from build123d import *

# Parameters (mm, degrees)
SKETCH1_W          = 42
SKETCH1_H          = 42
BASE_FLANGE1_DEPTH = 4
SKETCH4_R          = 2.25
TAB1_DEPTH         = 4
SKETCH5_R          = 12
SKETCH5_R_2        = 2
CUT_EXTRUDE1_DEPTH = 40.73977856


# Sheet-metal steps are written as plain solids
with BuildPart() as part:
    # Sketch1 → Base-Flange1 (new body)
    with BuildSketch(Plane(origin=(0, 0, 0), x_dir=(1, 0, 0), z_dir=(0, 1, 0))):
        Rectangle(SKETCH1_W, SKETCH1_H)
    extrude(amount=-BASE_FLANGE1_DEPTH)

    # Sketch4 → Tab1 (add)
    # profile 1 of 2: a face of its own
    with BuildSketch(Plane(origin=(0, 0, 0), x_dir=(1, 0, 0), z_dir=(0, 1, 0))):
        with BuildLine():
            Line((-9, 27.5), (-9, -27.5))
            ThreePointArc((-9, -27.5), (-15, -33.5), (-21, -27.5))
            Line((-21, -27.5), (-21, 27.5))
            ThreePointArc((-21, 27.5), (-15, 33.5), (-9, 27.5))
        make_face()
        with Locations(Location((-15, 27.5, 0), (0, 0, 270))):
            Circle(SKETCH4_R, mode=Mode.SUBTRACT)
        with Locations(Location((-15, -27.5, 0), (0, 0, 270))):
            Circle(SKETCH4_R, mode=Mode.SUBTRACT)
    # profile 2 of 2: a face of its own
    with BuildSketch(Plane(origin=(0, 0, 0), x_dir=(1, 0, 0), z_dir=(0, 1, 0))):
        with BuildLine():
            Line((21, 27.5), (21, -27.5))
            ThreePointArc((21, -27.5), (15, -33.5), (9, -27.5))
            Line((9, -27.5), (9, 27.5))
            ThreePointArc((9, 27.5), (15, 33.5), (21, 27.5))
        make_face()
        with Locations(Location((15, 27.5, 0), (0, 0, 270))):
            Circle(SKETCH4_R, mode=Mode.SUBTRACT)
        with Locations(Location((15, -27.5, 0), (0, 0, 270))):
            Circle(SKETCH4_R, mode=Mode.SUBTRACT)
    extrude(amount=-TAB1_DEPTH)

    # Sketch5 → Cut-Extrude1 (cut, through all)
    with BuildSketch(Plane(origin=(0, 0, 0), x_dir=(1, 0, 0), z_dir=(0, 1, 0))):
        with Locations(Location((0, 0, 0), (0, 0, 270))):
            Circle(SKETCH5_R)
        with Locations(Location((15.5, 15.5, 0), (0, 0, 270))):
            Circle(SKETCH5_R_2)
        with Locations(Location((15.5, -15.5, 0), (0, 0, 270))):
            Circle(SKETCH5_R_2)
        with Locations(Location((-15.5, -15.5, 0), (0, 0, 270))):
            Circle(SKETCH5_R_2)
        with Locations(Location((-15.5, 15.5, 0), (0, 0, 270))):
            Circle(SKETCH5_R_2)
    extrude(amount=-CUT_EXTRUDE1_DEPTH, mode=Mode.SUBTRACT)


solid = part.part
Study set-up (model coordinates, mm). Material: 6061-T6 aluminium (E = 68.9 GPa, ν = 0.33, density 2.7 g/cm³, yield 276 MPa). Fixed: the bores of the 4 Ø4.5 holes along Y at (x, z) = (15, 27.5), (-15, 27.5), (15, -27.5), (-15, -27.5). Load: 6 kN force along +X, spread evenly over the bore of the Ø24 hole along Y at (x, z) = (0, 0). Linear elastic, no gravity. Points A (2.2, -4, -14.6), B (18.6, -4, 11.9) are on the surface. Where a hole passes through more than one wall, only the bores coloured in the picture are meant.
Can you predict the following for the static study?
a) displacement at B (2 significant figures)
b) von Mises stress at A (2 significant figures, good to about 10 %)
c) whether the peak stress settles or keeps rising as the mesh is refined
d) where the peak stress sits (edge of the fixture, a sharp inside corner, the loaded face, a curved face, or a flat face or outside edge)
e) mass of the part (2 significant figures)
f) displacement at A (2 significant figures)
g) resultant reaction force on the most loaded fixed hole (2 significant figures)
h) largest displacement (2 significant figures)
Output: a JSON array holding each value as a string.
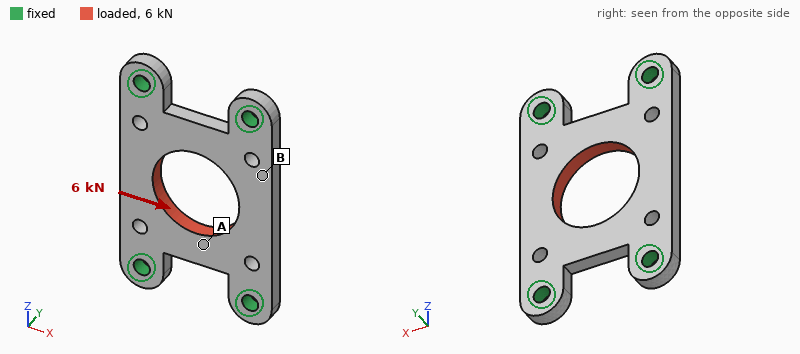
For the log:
["31 µm", "76 MPa", "keeps rising", "edge of the fixture", "19 g", "26 µm", "1.6 kN", "45 µm"]
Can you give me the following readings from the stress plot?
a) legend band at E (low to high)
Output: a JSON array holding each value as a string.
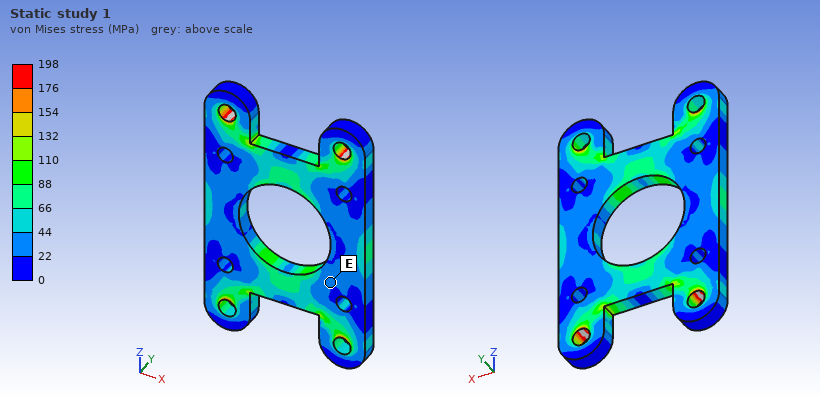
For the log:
["22 to 44 MPa"]
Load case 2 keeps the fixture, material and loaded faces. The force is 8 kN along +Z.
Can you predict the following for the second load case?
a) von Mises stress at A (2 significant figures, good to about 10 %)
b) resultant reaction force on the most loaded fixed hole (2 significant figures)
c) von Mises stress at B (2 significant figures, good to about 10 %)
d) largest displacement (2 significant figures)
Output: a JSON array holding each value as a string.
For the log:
["25 MPa", "2.1 kN", "32 MPa", "18 µm"]
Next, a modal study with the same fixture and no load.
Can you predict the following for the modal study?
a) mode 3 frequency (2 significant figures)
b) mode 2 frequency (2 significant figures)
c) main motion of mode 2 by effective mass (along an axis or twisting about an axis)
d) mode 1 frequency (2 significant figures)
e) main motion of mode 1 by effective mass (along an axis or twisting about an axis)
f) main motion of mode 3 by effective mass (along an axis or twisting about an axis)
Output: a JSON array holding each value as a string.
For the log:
["14 kHz", "8500 Hz", "twisting about Z", "6900 Hz", "along Y", "twisting about X"]
